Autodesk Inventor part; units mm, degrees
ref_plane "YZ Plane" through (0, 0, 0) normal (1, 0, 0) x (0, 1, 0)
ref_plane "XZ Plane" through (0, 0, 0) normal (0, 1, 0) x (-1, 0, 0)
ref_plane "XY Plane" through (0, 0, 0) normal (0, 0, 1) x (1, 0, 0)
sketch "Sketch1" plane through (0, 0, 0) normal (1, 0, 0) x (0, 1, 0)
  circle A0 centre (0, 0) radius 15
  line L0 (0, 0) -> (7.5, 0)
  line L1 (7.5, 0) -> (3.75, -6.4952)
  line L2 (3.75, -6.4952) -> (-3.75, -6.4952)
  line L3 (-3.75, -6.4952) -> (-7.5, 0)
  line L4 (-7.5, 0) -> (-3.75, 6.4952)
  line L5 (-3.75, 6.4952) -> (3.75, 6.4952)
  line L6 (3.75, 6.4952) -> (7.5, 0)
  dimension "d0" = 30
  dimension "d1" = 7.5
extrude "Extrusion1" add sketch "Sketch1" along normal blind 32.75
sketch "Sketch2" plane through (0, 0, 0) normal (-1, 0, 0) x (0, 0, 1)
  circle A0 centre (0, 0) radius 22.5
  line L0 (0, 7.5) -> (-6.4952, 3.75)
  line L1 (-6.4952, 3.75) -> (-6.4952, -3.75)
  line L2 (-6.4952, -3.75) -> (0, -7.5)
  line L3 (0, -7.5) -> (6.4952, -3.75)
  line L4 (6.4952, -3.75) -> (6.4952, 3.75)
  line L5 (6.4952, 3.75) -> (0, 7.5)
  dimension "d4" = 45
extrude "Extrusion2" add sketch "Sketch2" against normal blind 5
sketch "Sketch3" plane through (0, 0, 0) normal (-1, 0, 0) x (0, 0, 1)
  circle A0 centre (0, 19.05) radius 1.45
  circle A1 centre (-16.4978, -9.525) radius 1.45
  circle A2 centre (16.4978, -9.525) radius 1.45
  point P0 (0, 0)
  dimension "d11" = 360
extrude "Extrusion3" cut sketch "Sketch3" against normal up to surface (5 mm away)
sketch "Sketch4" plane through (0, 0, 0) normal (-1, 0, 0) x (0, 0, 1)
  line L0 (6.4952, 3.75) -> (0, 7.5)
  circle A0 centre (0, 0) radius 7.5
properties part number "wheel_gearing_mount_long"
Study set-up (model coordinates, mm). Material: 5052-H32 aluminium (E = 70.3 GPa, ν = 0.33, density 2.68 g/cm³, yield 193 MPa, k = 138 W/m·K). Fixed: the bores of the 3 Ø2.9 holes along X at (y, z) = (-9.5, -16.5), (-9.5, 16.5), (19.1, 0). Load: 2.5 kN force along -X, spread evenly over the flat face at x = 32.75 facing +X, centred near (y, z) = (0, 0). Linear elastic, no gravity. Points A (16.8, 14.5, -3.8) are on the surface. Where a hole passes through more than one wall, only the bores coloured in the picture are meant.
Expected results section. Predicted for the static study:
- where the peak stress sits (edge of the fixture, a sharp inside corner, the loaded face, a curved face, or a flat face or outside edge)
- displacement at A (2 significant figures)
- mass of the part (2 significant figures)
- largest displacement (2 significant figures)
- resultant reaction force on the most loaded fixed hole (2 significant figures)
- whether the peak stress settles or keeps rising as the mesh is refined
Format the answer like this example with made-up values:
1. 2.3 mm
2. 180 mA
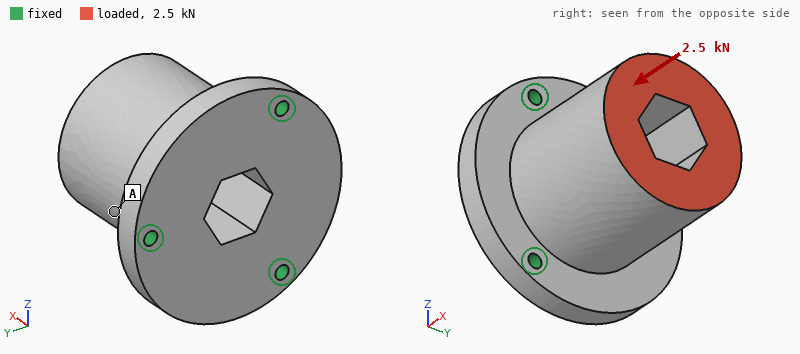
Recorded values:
1. edge of the fixture
2. 6.9 µm
3. 61 g
4. 8.0 µm
5. 880 N
6. keeps rising
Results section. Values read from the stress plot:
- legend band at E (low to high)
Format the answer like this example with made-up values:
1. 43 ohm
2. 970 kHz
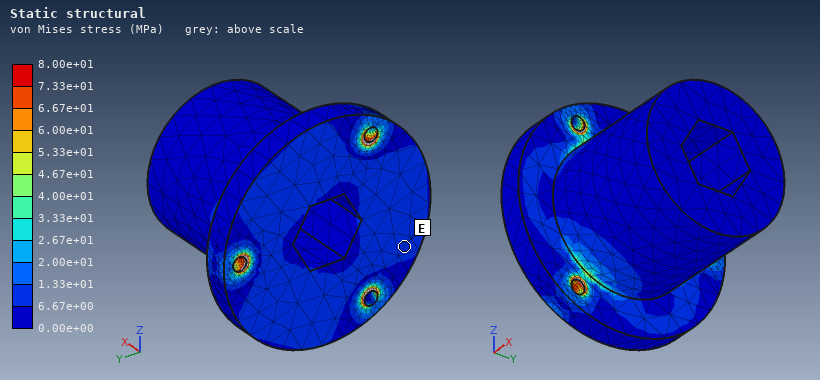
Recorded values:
1. 6.67e+00 to 1.33e+01 MPa
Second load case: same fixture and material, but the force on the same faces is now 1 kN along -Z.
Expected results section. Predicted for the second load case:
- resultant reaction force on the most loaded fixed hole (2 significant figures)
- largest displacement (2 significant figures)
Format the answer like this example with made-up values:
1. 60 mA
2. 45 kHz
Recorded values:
1. 1.1 kN
2. 24 µm
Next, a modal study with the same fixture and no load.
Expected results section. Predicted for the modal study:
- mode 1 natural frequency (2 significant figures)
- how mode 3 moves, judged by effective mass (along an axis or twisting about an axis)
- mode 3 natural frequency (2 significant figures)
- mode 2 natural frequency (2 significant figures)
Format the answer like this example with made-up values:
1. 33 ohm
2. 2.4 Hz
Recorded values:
1. 8200 Hz
2. along X
3. 13 kHz
4. 8200 Hz
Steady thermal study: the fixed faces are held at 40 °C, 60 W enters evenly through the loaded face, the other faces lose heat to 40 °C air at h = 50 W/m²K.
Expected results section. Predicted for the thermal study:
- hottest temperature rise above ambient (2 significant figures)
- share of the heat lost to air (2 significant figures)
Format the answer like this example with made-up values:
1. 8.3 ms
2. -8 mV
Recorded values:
1. 34 K
2. 9.9 %
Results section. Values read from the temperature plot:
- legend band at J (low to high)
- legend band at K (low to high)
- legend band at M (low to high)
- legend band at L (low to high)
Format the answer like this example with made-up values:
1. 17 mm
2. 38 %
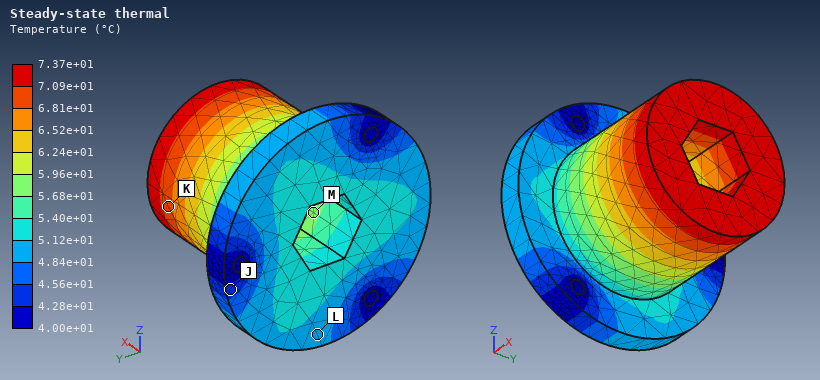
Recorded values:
1. 4.28e+01 to 4.56e+01 °C
2. 6.81e+01 to 7.09e+01 °C
3. 5.68e+01 to 5.96e+01 °C
4. 4.84e+01 to 5.12e+01 °C
